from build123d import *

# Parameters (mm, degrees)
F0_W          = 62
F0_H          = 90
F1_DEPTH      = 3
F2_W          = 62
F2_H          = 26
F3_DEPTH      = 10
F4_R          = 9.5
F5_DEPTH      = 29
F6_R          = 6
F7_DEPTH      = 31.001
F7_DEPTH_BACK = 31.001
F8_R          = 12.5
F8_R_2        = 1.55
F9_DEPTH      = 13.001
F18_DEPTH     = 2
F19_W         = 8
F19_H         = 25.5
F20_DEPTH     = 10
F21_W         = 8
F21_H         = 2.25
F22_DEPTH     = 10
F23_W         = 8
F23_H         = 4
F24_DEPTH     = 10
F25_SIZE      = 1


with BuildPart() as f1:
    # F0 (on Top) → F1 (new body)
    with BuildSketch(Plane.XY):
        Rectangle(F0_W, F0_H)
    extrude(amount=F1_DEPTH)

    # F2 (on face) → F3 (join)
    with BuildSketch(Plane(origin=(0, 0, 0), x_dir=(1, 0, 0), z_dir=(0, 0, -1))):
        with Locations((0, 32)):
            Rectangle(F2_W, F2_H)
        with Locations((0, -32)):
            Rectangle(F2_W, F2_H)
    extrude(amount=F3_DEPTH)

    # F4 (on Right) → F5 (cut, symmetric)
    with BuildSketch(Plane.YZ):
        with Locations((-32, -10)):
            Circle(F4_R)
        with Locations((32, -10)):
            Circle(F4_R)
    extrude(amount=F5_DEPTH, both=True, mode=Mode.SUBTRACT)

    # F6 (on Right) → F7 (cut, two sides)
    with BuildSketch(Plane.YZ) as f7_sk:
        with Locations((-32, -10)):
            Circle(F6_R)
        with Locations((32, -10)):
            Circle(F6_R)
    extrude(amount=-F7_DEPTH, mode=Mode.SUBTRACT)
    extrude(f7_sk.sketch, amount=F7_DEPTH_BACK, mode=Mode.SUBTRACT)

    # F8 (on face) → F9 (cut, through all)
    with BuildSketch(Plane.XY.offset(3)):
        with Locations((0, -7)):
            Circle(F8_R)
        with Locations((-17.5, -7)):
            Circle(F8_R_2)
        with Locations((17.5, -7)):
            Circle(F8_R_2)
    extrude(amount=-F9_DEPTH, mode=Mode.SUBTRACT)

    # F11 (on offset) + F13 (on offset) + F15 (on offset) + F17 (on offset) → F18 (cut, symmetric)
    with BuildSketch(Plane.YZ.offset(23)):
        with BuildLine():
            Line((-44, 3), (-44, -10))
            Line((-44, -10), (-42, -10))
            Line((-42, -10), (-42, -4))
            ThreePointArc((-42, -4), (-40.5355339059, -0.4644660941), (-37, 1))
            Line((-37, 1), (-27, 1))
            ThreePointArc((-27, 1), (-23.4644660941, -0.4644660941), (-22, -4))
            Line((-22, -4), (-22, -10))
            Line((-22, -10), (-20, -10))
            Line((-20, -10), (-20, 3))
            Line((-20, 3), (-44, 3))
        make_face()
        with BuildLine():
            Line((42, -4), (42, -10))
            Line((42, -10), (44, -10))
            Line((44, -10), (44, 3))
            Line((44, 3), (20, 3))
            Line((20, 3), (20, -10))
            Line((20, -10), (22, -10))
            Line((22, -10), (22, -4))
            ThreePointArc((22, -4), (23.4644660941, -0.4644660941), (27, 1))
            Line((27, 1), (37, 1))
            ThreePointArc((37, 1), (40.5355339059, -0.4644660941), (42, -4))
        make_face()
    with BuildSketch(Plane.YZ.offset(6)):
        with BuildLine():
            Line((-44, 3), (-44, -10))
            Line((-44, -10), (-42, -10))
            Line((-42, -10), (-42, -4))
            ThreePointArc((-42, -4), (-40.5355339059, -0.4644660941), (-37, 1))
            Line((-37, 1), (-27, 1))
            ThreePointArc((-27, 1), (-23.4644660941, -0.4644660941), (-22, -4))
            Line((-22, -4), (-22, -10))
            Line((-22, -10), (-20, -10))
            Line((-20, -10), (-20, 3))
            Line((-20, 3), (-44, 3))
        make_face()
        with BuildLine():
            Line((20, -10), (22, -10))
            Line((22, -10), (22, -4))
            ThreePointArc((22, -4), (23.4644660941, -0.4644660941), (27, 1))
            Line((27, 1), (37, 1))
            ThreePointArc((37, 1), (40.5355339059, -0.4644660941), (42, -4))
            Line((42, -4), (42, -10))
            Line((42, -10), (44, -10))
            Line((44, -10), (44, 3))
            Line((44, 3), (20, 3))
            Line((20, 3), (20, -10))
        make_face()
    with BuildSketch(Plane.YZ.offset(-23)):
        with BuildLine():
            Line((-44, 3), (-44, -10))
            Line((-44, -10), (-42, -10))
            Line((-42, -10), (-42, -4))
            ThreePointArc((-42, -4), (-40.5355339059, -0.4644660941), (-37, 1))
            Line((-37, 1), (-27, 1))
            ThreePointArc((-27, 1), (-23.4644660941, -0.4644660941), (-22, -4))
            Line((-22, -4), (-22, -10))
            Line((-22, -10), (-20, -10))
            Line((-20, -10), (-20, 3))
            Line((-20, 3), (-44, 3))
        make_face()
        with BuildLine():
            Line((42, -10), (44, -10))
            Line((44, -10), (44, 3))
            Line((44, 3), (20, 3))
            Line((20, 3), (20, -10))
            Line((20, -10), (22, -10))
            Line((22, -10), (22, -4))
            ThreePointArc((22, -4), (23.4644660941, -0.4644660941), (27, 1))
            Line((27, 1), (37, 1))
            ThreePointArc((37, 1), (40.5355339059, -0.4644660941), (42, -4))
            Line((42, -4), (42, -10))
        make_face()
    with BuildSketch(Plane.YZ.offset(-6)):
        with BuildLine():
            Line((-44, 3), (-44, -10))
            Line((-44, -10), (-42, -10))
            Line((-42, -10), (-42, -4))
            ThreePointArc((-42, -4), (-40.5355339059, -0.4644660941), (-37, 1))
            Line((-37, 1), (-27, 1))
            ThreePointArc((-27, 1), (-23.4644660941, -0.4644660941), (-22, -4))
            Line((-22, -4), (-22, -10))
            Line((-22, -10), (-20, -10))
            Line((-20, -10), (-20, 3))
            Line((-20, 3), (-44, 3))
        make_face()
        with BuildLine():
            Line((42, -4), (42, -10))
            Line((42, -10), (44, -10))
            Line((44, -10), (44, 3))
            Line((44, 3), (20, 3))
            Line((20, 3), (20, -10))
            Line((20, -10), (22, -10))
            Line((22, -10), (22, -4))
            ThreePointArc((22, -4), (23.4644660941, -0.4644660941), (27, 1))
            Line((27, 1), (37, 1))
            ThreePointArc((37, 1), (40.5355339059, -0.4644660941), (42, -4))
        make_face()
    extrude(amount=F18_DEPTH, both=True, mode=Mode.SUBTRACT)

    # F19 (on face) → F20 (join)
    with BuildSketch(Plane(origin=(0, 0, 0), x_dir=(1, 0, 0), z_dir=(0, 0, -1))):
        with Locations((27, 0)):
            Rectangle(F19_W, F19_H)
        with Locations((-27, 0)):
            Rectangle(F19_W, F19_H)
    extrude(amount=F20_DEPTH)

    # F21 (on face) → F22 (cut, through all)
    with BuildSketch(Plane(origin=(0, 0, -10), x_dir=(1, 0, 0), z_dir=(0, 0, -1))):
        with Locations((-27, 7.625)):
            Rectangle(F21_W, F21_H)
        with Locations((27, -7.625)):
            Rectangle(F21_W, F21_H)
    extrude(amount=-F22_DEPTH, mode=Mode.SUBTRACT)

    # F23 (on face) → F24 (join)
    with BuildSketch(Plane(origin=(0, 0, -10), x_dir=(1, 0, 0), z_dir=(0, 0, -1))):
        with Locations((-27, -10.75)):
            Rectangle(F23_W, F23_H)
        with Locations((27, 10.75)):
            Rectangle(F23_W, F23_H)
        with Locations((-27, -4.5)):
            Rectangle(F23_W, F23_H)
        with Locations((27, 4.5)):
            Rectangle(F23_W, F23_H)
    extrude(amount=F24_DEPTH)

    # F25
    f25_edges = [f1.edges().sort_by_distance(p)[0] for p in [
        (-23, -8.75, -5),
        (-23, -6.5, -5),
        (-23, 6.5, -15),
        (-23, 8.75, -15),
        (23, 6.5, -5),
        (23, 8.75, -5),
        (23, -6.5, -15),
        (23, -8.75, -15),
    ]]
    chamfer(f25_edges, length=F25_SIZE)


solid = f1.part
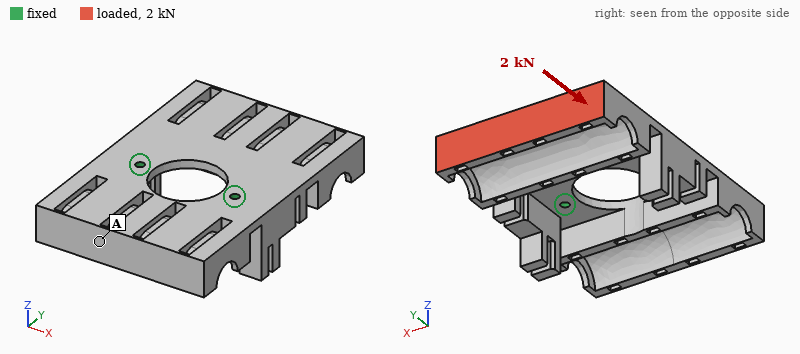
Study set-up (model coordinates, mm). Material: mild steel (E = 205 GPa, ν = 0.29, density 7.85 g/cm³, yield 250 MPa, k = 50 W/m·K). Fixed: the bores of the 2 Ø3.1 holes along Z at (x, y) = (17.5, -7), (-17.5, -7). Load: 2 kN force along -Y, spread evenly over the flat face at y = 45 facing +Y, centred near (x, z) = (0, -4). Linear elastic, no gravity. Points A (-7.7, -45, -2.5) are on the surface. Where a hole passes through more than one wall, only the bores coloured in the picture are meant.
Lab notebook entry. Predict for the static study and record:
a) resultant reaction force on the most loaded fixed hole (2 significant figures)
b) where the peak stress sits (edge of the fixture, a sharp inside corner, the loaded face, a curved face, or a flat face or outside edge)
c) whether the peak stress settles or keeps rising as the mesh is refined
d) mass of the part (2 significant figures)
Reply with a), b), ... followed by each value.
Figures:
a) 1.0 kN
b) edge of the fixture
c) keeps rising
d) 250 g
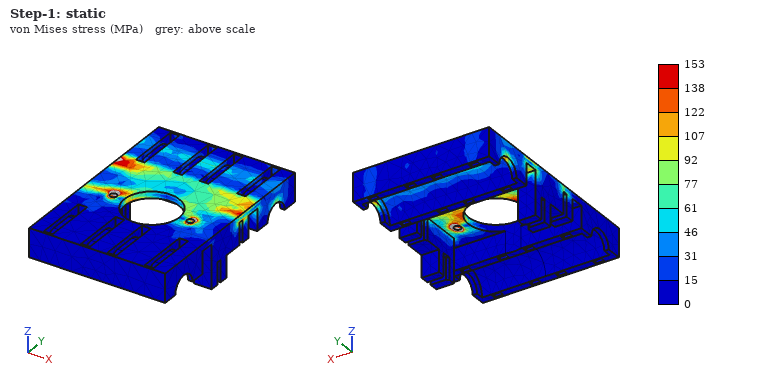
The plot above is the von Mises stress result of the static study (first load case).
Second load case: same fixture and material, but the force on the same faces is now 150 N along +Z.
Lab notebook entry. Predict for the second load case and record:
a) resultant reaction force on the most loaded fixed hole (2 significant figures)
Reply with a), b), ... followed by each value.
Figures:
a) 77 N
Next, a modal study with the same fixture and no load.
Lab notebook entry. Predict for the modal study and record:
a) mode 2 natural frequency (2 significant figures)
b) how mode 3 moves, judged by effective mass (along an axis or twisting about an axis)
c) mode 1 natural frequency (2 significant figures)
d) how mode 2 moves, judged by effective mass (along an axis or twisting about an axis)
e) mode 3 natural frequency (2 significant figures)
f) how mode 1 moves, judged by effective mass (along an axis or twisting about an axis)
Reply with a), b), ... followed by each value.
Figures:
a) 1000 Hz
b) twisting about Y
c) 620 Hz
d) along Z
e) 1700 Hz
f) along Z
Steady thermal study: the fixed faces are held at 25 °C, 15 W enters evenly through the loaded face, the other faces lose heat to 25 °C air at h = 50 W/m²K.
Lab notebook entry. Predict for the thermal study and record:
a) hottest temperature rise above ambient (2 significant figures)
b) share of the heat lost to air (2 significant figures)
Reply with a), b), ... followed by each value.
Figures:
a) 39 K
b) 75 %
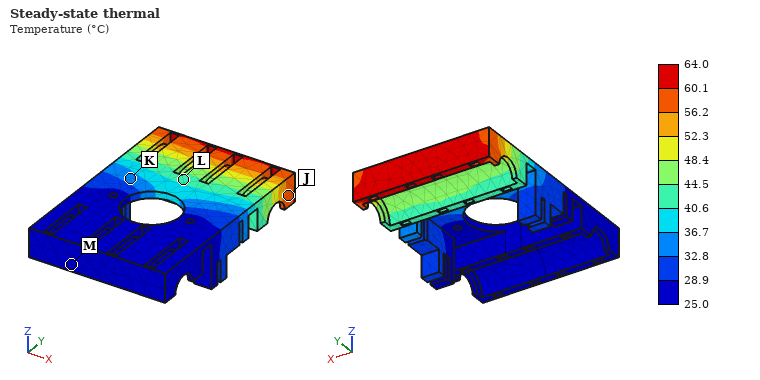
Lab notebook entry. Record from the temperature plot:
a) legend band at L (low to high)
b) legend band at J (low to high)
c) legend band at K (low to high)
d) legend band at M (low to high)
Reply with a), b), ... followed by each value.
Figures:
a) 40.6 to 44.5 °C
b) 56.2 to 60.1 °C
c) 32.8 to 36.7 °C
d) 25.0 to 28.9 °C
